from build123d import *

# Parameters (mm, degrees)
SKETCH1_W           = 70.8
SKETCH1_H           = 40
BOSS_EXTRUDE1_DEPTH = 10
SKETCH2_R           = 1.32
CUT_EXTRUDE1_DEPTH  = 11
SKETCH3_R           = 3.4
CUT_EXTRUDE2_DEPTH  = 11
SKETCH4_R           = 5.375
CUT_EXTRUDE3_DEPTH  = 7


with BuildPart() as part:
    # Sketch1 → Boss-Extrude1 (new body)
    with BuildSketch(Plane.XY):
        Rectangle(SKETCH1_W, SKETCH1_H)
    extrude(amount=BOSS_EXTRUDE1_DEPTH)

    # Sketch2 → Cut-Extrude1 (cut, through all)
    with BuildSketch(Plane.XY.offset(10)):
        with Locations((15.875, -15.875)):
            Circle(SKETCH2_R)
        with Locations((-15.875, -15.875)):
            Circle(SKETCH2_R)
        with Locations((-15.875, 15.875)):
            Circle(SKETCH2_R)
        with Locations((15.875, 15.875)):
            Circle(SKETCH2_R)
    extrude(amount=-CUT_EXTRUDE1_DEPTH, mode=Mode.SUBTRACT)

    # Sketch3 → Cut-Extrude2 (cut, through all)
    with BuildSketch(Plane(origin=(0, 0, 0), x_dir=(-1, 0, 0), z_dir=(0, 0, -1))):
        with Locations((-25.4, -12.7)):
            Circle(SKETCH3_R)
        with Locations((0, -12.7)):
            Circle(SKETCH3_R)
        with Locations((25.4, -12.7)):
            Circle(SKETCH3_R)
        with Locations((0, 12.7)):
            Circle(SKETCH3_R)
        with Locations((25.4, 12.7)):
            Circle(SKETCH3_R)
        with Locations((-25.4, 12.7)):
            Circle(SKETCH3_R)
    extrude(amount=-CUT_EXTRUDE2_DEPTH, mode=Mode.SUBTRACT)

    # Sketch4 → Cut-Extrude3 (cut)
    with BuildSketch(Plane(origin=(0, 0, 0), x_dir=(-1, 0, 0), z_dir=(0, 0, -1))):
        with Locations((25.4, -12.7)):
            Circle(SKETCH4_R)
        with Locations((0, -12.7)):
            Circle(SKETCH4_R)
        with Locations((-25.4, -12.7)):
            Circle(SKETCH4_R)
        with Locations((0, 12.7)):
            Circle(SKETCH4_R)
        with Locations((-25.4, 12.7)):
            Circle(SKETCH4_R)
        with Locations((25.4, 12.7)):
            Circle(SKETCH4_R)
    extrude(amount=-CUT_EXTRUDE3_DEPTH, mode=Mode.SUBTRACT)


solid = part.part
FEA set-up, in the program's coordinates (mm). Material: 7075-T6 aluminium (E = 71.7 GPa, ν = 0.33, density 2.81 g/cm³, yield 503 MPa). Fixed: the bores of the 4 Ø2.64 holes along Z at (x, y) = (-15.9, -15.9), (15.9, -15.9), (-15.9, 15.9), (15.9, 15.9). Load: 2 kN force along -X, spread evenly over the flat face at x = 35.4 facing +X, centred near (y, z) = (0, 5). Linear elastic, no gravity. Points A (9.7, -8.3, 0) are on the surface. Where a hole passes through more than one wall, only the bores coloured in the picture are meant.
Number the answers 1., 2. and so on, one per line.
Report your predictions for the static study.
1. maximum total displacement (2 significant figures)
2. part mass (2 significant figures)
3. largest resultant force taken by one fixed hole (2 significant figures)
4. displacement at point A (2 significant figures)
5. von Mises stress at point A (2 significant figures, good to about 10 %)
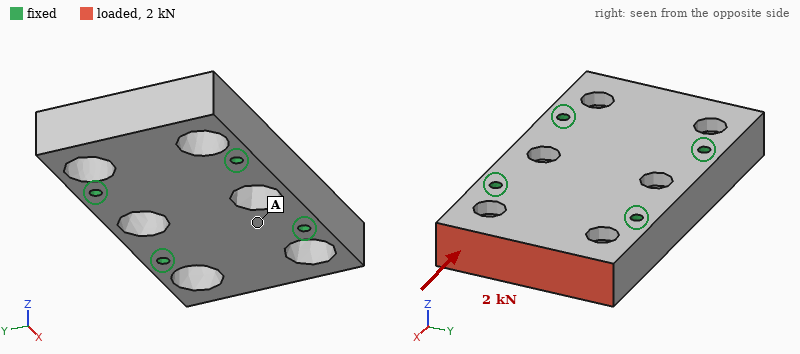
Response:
1. 5.3 µm
2. 66 g
3. 800 N
4. 1.1 µm
5. 3.2 MPa
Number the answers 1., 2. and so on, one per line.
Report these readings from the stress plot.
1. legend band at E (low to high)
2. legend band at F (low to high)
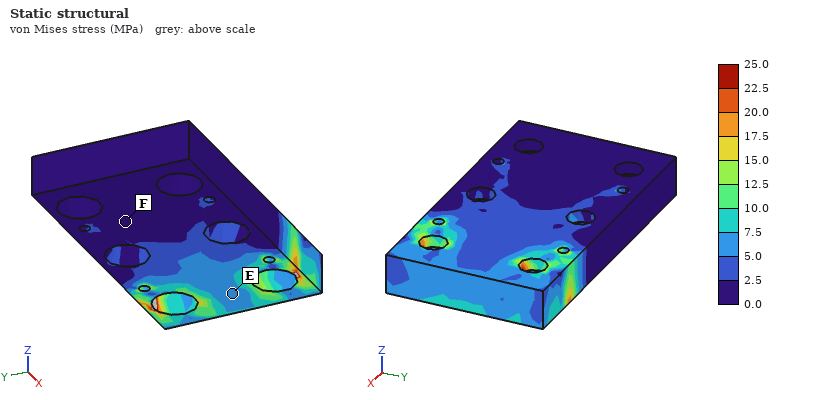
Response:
1. 5.0 to 7.5 MPa
2. 0.0 to 2.5 MPa
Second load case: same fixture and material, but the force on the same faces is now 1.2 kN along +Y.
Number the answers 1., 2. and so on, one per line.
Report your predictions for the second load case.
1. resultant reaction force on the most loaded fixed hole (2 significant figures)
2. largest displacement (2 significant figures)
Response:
1. 900 N
2. 7.6 µm
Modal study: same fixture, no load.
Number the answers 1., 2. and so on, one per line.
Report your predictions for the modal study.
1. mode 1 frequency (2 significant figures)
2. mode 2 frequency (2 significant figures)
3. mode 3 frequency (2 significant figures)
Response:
1. 12 kHz
2. 12 kHz
3. 20 kHz
